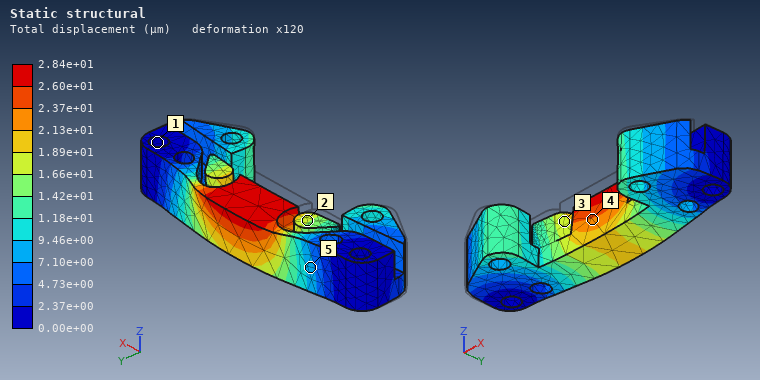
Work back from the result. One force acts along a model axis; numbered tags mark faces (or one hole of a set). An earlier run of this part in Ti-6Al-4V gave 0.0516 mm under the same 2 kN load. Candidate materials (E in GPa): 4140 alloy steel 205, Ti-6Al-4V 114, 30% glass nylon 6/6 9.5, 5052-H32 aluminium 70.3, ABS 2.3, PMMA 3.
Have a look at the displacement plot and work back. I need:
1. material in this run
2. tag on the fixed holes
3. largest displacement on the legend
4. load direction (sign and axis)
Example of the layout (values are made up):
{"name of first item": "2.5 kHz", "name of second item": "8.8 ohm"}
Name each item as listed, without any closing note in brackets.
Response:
{"material in this run": "4140 alloy steel", "tag on the fixed holes": "1", "largest displacement on the legend": "2.84e+01 µm", "load direction": "+Y"}
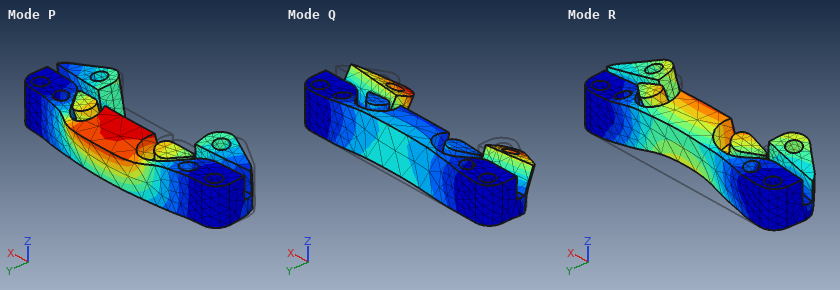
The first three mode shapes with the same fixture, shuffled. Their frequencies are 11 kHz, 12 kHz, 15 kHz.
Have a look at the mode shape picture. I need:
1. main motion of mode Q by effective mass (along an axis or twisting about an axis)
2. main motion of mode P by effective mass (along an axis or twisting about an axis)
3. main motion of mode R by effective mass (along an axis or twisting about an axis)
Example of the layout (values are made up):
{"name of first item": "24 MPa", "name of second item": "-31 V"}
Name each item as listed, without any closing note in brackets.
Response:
{"main motion of mode Q by effective mass": "twisting about X", "main motion of mode P by effective mass": "along Y", "main motion of mode R by effective mass": "along Z"}
